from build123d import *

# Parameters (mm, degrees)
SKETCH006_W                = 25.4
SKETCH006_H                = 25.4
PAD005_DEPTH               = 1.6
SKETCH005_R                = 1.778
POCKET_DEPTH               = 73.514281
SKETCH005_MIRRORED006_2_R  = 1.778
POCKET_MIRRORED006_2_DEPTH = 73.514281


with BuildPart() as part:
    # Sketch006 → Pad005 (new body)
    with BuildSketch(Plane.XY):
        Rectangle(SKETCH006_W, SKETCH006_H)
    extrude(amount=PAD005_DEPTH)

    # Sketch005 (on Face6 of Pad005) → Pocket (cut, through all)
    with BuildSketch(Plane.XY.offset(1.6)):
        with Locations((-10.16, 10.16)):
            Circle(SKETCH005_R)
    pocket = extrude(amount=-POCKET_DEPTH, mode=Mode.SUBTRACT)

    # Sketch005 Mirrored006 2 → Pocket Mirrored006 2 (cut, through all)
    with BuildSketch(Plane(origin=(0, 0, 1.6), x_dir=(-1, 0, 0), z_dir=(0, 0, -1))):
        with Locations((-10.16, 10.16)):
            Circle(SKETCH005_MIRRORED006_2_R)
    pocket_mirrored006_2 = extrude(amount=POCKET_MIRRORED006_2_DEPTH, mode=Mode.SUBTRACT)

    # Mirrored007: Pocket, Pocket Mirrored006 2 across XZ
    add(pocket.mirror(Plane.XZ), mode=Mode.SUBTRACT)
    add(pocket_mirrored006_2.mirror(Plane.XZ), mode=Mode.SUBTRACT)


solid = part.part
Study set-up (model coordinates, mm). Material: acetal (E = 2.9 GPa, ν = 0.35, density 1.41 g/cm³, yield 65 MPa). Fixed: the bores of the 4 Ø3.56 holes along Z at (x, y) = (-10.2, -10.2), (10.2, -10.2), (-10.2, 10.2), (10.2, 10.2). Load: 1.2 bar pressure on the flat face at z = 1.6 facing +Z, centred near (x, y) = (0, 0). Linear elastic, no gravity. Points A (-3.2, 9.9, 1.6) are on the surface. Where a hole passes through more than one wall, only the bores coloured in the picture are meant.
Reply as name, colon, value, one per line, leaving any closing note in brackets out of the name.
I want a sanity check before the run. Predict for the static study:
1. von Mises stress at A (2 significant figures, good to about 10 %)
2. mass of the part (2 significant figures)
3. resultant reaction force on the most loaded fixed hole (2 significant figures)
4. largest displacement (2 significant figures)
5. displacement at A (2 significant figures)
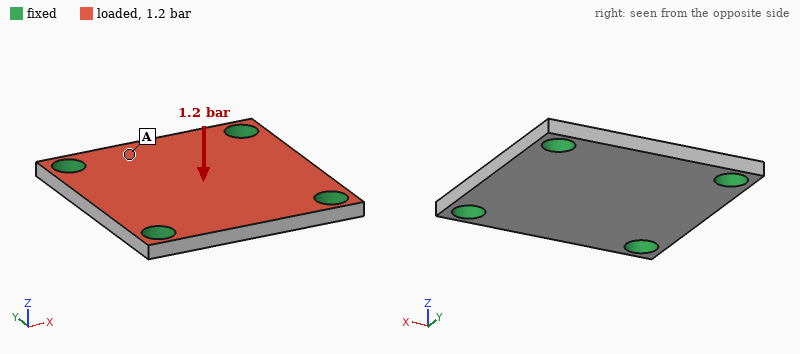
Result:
von Mises stress at A: 3.0 MPa
mass of the part: 1.4 g
resultant reaction force on the most loaded fixed hole: 18 N
largest displacement: 87 µm
displacement at A: 35 µm
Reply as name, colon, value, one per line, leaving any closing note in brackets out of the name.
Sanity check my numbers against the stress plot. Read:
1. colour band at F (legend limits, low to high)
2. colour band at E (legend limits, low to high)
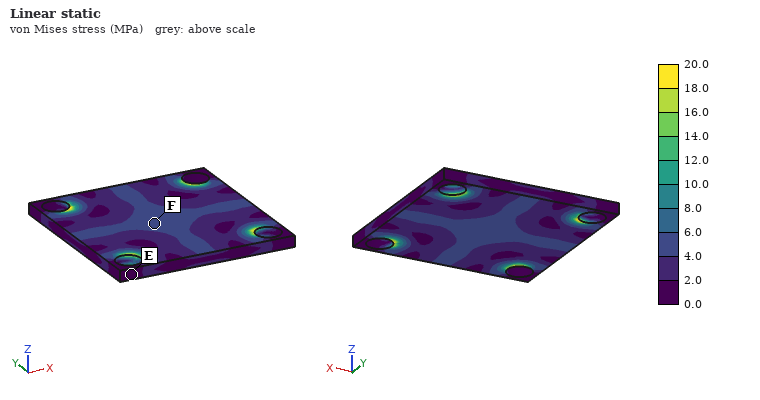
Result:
colour band at F: 4.0 to 6.0 MPa
colour band at E: 0.0 to 2.0 MPa
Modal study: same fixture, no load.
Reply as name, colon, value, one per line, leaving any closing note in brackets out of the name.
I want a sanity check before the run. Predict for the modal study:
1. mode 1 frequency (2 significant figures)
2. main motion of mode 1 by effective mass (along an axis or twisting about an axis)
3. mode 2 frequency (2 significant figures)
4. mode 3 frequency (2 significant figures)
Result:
mode 1 frequency: 4800 Hz
main motion of mode 1 by effective mass: along Z
mode 2 frequency: 7800 Hz
mode 3 frequency: 7800 Hz
